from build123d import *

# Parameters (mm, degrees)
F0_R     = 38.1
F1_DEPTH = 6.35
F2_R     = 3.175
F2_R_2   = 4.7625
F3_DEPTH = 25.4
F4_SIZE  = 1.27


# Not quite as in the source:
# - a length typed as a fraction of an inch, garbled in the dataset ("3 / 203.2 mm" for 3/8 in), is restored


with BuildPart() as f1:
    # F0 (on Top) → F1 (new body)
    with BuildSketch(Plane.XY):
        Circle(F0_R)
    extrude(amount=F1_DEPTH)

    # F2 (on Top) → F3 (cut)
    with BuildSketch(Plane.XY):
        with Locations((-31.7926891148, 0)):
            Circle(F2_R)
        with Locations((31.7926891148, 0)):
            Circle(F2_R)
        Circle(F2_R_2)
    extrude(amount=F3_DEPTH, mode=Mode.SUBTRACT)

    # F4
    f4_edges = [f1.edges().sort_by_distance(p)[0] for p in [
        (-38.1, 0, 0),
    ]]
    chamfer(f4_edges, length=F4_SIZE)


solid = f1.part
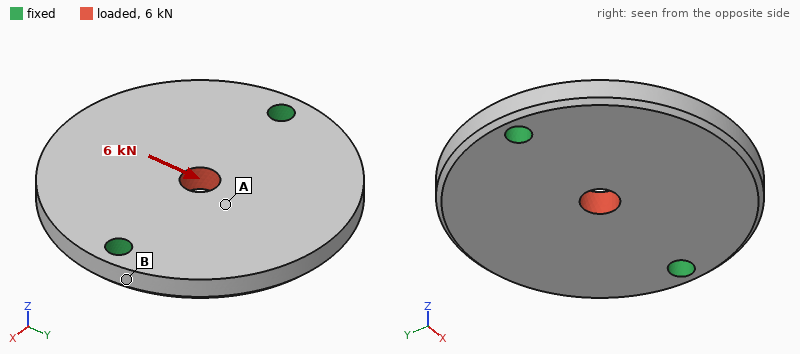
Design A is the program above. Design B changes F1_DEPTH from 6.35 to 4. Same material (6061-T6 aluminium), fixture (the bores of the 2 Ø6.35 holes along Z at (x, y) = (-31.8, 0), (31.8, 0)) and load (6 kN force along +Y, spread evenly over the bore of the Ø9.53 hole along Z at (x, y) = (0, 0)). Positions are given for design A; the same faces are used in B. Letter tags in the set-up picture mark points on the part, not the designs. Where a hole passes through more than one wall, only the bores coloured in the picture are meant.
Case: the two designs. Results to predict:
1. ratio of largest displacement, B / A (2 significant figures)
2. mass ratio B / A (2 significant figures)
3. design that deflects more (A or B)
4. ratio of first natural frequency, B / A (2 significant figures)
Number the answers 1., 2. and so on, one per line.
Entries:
1. 1.6
2. 0.63
3. B
4. 0.67
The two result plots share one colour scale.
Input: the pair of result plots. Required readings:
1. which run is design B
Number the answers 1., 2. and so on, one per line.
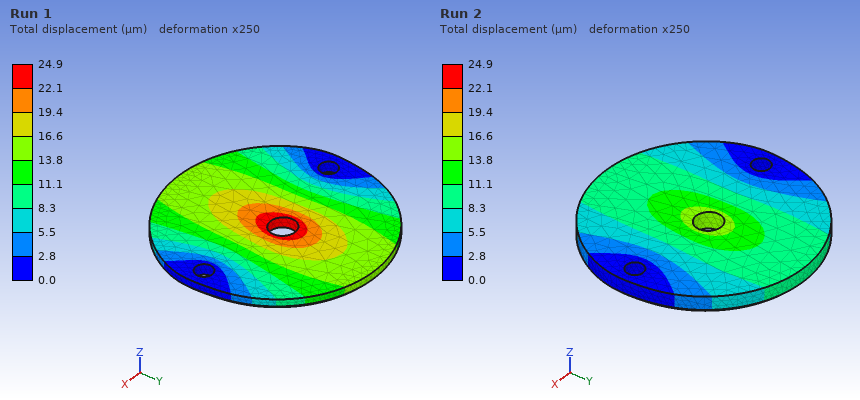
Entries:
1. Run 1
